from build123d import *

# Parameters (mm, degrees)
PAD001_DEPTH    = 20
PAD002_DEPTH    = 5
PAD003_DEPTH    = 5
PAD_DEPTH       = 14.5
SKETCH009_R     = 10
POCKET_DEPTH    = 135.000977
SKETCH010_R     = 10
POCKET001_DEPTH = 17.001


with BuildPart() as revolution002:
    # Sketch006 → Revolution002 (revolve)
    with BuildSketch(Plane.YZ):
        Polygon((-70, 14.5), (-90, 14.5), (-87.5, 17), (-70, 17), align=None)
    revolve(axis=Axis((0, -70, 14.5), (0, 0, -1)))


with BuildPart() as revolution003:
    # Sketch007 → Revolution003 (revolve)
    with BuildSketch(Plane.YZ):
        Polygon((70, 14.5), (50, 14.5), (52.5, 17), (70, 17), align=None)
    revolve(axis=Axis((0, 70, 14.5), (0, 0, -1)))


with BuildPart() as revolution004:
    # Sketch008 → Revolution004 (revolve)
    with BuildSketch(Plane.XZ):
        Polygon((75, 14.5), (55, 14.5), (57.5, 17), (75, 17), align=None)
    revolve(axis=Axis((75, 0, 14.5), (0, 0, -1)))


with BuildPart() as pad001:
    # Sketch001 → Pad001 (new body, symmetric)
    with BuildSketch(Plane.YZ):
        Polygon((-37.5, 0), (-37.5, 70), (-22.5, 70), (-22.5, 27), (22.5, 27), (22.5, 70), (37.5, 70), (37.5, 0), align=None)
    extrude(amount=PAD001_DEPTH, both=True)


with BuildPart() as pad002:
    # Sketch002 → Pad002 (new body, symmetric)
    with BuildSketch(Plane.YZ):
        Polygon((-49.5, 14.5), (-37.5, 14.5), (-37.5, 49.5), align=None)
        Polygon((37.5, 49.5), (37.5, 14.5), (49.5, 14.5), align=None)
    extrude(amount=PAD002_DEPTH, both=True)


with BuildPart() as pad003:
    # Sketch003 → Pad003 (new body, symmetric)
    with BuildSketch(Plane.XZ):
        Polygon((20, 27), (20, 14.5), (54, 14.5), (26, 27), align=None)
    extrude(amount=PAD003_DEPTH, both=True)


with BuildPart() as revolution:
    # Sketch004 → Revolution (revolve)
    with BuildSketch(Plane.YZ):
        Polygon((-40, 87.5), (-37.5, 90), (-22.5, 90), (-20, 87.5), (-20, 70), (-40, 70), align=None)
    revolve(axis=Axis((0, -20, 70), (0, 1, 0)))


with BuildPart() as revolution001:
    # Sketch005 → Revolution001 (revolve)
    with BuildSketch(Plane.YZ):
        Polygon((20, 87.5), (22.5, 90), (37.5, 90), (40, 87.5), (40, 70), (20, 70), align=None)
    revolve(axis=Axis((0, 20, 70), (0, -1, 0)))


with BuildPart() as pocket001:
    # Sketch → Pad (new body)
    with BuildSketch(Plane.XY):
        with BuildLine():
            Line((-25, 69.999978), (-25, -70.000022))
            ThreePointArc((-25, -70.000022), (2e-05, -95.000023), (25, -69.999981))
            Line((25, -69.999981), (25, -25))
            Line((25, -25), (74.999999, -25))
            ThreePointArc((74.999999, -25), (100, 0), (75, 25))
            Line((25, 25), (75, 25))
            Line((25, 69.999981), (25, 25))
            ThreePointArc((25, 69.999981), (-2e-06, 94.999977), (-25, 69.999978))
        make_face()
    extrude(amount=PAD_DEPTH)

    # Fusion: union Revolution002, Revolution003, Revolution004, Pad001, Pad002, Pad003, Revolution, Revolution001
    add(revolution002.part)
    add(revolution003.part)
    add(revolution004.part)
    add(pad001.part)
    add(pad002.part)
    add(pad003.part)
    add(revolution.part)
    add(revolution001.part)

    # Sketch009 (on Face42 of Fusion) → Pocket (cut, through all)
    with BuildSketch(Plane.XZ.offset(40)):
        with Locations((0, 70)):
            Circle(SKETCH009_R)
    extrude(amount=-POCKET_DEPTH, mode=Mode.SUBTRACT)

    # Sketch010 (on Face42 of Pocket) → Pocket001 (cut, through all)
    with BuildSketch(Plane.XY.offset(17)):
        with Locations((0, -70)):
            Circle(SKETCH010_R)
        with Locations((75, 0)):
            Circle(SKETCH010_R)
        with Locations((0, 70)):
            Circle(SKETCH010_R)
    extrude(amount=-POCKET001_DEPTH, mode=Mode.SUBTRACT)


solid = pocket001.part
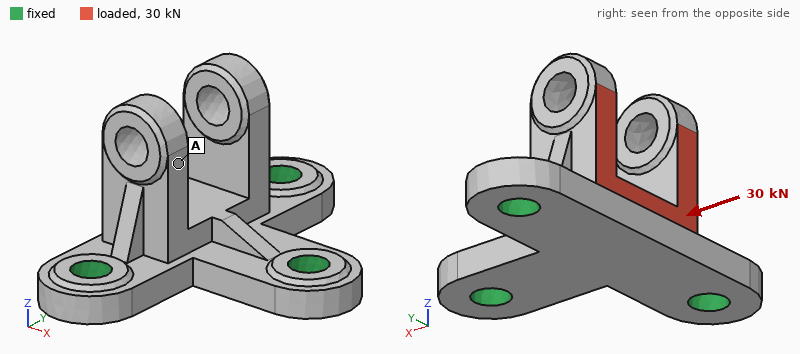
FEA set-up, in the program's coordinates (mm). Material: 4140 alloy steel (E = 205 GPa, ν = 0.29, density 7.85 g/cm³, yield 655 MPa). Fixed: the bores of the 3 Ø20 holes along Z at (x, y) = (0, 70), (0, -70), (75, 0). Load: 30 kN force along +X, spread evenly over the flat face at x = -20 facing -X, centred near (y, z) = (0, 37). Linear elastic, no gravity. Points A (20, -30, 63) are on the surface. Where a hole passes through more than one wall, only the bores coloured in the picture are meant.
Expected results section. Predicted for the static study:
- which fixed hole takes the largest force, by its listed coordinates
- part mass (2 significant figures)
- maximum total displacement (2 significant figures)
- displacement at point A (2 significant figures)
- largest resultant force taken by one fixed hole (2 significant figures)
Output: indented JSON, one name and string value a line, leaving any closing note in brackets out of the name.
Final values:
{
  "which fixed hole takes the largest force, by its listed coordinates": "(75, 0)",
  "part mass": "2.2 kg",
  "maximum total displacement": "0.13 mm",
  "displacement at point A": "0.089 mm",
  "largest resultant force taken by one fixed hole": "20 kN"
}
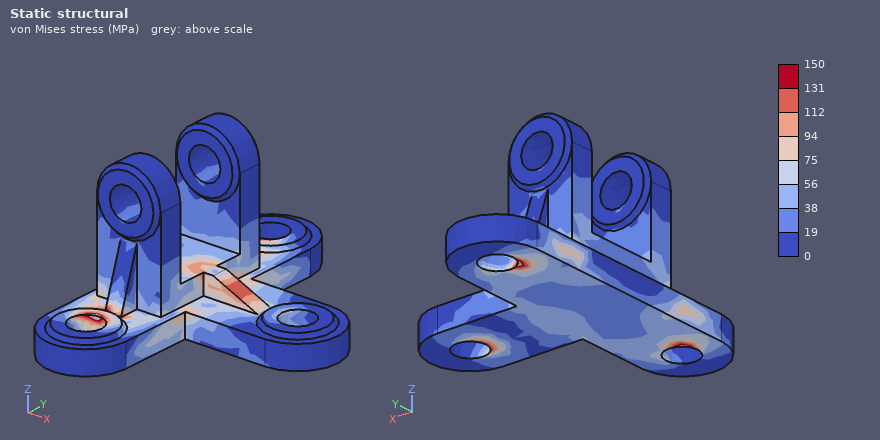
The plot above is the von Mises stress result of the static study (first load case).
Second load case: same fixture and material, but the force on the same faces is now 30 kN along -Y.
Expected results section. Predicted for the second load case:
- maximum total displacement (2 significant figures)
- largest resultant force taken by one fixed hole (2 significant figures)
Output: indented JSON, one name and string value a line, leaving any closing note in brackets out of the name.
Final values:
{
  "maximum total displacement": "0.10 mm",
  "largest resultant force taken by one fixed hole": "18 kN"
}
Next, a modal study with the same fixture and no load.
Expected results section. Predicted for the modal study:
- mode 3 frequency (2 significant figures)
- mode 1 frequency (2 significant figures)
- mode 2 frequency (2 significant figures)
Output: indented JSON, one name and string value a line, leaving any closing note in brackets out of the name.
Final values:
{
  "mode 3 frequency": "3100 Hz",
  "mode 1 frequency": "2600 Hz",
  "mode 2 frequency": "3000 Hz"
}
